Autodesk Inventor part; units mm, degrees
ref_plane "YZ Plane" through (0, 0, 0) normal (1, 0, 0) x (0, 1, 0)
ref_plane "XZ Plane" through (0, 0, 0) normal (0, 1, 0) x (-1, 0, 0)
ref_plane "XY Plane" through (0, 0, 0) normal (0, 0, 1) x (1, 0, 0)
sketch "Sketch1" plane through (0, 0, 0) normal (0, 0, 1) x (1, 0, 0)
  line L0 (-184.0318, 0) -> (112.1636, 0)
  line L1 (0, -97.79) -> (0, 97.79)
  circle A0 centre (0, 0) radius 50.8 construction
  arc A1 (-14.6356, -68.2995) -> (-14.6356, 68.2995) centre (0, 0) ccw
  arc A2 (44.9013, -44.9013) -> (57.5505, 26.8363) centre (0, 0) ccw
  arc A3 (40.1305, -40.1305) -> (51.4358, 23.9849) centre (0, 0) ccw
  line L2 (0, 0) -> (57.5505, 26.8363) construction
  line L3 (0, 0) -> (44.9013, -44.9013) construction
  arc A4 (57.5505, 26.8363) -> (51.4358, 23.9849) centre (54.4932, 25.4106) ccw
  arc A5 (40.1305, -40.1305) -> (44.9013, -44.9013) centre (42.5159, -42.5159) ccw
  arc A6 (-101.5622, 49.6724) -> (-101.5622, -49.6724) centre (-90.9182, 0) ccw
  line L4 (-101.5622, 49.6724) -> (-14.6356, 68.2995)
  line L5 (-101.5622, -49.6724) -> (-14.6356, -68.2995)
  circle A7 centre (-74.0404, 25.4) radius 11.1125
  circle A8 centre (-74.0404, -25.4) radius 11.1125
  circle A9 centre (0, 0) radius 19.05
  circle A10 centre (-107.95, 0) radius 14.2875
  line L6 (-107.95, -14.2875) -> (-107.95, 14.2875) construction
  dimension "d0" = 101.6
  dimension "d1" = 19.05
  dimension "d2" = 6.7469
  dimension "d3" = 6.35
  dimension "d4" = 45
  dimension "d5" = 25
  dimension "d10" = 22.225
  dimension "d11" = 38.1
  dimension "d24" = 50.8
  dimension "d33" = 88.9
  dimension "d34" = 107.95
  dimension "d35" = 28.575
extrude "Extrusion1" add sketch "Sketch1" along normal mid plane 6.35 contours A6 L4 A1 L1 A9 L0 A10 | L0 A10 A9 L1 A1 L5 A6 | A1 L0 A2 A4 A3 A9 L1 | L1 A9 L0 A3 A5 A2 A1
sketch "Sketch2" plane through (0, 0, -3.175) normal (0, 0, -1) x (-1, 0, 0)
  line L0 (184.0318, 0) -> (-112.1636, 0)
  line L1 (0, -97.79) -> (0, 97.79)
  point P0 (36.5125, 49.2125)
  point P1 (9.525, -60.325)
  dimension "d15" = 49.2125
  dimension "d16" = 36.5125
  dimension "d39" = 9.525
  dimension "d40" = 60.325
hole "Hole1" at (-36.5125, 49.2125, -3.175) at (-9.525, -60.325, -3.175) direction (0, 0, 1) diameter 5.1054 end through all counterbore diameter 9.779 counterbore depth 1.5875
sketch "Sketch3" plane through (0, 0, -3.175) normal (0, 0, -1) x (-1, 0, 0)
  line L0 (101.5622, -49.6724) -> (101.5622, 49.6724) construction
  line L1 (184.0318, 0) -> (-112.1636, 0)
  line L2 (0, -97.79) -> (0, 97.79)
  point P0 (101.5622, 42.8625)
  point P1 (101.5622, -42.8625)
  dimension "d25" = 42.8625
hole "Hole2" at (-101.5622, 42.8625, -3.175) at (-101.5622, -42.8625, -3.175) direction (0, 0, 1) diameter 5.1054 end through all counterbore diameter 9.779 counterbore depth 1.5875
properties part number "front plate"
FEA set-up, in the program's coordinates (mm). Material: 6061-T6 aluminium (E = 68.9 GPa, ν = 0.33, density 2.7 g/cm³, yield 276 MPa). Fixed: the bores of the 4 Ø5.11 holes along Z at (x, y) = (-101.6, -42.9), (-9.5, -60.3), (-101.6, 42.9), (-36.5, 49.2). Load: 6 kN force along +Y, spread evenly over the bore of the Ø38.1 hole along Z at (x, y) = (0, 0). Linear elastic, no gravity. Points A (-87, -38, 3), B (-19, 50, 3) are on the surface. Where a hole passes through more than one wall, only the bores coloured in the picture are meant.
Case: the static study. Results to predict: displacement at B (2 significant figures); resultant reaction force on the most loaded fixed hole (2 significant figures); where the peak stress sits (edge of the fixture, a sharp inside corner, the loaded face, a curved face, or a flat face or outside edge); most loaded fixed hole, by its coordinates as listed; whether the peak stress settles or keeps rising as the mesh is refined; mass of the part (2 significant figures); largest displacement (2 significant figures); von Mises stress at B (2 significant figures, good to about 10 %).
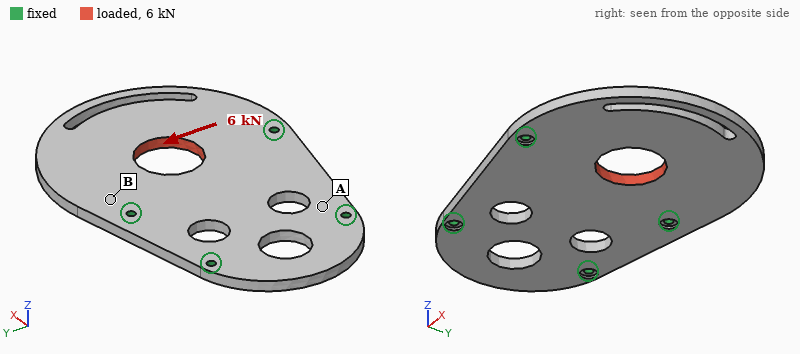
8.9 µm
3.3 kN
edge of the fixture
(-9.5, -60.3)
keeps rising
340 g
24 µm
10 MPa
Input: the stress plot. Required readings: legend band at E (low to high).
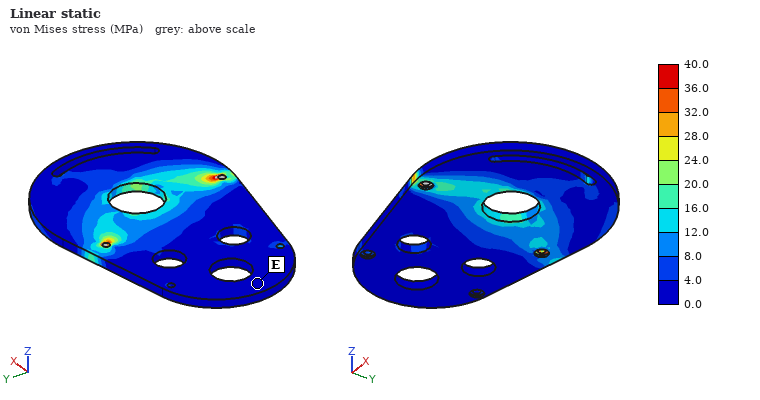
0.0 to 4.0 MPa
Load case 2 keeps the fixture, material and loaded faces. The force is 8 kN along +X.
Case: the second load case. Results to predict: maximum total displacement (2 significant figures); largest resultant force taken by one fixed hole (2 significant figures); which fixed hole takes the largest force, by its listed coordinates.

26 µm
3.3 kN
(-36.5, 49.2)
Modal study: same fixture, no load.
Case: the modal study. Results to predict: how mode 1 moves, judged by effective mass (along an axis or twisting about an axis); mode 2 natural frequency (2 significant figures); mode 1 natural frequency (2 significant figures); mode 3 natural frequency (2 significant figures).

along Z
1500 Hz
590 Hz
2100 Hz
